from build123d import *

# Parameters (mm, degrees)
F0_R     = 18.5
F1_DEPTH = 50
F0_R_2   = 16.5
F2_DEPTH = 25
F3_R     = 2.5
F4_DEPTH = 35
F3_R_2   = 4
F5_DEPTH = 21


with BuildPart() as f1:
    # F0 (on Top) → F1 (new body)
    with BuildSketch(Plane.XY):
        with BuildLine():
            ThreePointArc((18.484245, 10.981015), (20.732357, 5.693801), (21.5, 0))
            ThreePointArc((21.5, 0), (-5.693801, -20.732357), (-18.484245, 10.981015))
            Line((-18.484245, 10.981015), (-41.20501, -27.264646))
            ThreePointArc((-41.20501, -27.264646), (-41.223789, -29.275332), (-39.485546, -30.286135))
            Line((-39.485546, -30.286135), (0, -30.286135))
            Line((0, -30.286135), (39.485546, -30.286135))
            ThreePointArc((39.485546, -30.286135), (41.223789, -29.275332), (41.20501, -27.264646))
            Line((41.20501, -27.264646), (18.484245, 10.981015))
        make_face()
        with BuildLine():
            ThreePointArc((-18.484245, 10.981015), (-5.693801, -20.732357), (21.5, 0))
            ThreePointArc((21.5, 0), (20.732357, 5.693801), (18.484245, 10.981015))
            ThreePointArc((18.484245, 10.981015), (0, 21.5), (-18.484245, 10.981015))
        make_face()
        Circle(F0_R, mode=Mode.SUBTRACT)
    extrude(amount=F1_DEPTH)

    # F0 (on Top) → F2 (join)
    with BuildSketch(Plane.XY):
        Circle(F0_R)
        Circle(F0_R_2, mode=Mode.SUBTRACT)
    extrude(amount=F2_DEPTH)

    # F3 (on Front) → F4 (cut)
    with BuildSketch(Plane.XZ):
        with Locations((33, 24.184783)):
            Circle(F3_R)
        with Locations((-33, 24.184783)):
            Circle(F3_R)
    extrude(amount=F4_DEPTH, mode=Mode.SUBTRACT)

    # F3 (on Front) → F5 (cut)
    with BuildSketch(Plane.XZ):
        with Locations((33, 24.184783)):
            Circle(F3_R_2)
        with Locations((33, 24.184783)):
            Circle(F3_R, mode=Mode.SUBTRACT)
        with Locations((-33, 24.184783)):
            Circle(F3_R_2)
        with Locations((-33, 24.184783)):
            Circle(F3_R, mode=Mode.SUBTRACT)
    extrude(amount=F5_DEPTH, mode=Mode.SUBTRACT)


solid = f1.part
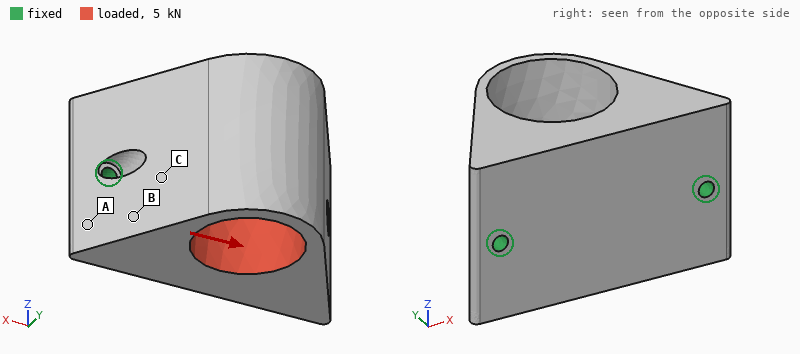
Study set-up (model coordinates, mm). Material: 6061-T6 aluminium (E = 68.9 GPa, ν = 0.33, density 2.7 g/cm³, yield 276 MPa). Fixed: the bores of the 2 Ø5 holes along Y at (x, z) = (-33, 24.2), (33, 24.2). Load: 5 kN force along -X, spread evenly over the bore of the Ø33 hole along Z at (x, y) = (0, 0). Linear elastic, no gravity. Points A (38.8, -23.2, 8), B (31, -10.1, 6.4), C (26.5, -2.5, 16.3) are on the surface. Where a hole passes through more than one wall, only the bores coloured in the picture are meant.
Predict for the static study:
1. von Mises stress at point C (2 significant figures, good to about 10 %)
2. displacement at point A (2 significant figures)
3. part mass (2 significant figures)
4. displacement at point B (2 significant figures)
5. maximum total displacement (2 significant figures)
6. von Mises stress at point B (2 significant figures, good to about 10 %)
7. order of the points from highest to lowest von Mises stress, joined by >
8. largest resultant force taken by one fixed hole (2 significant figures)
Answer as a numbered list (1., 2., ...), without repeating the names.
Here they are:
1. 18 MPa
2. 4.8 µm
3. 250 g
4. 7.1 µm
5. 31 µm
6. 11 MPa
7. C > B > A
8. 3.2 kN
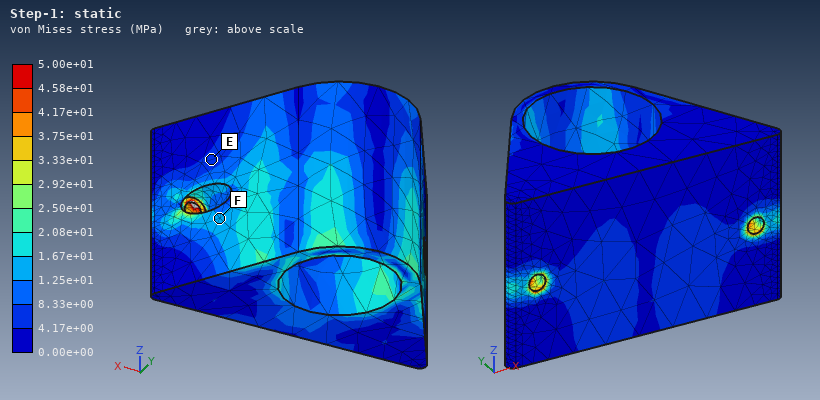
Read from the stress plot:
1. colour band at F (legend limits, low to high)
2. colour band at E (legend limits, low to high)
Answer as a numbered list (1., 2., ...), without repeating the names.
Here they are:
1. 1.25e+01 to 1.67e+01 MPa
2. 4.17e+00 to 8.33e+00 MPa
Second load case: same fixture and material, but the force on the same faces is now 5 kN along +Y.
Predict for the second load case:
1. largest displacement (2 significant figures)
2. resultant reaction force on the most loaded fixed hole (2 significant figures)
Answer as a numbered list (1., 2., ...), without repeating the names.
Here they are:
1. 72 µm
2. 2.7 kN
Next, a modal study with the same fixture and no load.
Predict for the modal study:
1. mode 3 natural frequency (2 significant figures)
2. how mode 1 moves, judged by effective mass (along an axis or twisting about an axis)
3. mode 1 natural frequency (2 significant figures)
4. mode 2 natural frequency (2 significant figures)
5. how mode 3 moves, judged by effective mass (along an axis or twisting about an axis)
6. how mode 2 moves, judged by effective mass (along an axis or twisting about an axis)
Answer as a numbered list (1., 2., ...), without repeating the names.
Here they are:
1. 8600 Hz
2. along Z
3. 3100 Hz
4. 7600 Hz
5. along X
6. along Y
